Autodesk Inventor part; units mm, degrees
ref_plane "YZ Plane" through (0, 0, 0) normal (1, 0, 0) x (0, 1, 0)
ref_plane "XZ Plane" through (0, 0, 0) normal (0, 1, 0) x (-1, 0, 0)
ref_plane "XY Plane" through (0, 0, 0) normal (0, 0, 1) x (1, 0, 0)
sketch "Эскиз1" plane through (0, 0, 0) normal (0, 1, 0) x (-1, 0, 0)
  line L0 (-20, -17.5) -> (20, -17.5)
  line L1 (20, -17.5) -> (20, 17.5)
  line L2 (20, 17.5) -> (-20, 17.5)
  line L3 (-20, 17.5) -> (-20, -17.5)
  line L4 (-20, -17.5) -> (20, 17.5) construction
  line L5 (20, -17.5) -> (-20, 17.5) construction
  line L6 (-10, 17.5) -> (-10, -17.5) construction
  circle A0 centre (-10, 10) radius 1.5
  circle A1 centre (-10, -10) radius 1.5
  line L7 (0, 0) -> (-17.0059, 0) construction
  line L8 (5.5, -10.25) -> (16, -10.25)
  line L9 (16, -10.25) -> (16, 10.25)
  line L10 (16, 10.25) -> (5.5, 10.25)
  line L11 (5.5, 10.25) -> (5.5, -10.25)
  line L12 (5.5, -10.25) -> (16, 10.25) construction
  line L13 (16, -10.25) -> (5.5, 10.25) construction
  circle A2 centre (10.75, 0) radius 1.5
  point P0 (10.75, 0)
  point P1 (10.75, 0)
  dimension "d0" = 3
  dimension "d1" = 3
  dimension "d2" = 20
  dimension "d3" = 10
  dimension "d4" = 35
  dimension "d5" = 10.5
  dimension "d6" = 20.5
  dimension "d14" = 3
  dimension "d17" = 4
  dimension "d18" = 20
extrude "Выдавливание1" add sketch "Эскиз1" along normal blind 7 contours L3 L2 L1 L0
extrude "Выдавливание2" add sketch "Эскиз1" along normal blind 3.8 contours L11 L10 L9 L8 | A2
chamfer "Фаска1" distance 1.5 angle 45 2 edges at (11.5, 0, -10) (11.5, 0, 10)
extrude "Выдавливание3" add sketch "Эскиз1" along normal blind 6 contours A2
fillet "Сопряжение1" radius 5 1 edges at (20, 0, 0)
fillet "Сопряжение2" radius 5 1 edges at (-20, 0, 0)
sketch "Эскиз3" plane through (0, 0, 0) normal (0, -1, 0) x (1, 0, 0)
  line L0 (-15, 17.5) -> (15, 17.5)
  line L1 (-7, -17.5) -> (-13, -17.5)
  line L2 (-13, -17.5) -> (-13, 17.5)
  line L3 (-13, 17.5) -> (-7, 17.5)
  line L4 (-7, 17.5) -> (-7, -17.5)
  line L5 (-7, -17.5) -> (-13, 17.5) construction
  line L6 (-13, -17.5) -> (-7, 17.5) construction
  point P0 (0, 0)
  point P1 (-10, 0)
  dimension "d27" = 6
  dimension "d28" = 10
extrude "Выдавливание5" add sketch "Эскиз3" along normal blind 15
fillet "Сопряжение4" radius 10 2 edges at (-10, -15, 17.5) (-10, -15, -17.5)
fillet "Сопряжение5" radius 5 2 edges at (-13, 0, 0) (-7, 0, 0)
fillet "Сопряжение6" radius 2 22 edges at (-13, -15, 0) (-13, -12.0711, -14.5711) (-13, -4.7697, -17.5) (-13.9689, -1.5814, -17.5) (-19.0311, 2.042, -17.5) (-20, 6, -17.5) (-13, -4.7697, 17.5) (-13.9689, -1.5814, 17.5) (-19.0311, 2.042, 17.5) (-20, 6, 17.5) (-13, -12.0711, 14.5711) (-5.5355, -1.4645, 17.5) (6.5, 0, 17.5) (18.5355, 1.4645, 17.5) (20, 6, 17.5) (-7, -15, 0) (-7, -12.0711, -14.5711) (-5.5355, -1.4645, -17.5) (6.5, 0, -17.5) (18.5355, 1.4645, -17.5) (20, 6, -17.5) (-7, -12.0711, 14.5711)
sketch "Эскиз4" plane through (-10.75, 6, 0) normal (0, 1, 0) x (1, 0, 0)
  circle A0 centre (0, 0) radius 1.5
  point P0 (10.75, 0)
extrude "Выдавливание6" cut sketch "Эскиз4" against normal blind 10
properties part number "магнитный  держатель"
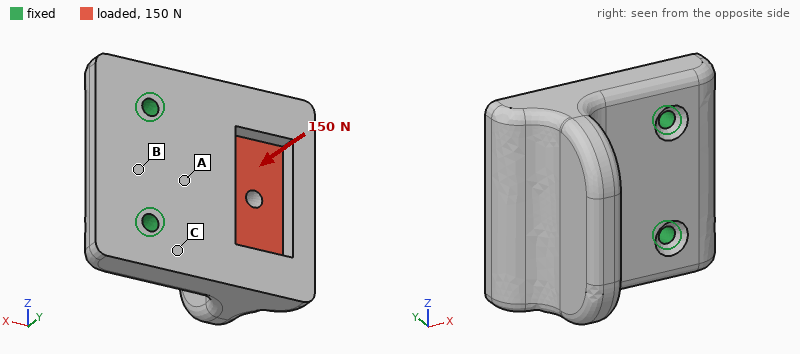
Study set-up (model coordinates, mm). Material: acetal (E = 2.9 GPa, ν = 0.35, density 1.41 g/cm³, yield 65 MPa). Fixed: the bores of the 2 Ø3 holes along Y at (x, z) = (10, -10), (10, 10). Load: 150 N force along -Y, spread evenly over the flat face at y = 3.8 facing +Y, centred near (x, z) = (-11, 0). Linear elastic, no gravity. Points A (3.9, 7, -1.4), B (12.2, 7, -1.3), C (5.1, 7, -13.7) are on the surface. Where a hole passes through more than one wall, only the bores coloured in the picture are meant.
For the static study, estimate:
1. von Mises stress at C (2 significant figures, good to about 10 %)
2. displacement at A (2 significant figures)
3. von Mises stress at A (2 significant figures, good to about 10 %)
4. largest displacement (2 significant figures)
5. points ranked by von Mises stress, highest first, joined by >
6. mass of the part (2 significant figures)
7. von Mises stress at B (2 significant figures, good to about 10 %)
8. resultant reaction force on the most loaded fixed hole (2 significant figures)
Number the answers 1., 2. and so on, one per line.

1. 8.5 MPa
2. 0.061 mm
3. 5.6 MPa
4. 0.40 mm
5. C > A > B
6. 16 g
7. 2.8 MPa
8. 75 N
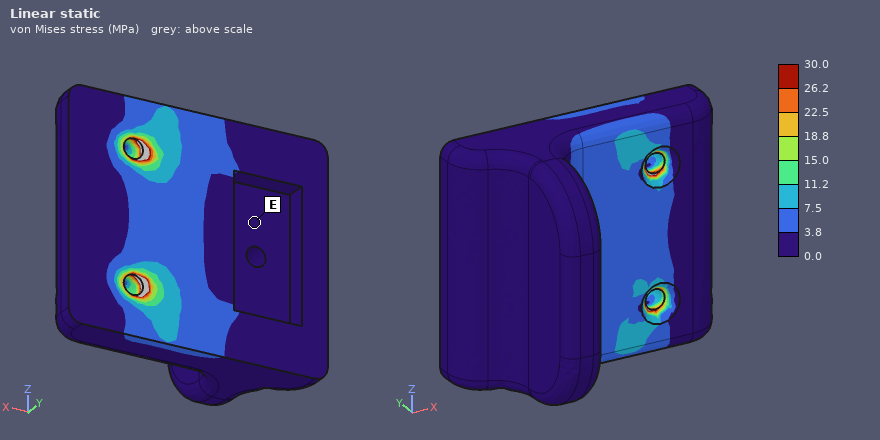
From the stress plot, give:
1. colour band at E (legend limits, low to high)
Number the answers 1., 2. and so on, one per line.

1. 0.0 to 3.8 MPa
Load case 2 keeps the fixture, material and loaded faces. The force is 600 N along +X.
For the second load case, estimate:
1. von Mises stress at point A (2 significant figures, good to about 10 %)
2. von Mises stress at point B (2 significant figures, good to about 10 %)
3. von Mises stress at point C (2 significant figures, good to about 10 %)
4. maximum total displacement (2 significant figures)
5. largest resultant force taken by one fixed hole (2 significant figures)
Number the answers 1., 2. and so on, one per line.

1. 2.1 MPa
2. 1.0 MPa
3. 2.9 MPa
4. 95 µm
5. 300 N
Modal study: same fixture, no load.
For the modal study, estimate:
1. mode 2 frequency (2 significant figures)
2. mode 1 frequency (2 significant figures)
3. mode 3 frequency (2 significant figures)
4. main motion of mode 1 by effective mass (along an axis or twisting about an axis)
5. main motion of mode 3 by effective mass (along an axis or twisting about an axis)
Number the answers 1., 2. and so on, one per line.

1. 2300 Hz
2. 1100 Hz
3. 3700 Hz
4. along Y
5. along Z
